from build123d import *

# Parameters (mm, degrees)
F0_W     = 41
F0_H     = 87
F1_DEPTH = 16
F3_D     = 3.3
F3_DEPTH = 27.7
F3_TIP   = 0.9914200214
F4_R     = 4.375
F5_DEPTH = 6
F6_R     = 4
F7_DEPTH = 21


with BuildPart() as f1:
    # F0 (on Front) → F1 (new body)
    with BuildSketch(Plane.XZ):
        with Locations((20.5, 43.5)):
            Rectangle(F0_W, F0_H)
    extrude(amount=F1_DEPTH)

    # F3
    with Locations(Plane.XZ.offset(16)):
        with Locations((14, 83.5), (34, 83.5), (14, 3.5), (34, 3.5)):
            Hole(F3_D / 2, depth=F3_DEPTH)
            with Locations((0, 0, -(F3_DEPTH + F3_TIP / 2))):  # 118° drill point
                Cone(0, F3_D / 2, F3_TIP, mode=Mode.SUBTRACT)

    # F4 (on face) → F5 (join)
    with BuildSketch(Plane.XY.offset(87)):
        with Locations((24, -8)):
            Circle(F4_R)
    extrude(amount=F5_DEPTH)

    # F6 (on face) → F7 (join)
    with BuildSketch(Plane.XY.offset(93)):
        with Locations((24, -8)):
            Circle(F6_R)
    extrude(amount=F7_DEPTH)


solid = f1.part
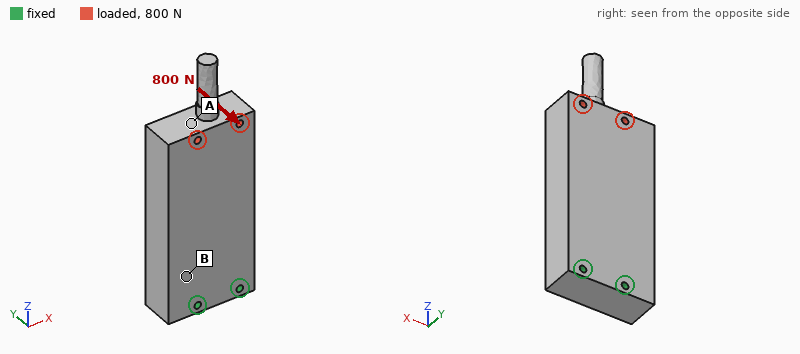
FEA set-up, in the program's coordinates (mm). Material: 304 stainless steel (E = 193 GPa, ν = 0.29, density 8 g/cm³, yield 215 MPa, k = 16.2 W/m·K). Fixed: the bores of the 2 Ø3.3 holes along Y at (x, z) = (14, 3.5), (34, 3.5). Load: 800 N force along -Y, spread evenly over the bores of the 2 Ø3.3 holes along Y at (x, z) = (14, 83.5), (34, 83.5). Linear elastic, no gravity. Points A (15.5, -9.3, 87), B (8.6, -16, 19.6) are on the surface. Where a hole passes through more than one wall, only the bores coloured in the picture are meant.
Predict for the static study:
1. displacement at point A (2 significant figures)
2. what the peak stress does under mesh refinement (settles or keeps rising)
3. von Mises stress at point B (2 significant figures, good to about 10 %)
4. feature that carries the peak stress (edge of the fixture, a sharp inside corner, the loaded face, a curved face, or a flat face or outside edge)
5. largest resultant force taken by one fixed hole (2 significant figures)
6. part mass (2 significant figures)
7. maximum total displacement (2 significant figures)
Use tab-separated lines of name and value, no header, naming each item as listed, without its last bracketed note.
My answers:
displacement at point A	66 µm
what the peak stress does under mesh refinement	keeps rising
von Mises stress at point B	27 MPa
feature that carries the peak stress	edge of the fixture
largest resultant force taken by one fixed hole	410 N
part mass	460 g
maximum total displacement	96 µm
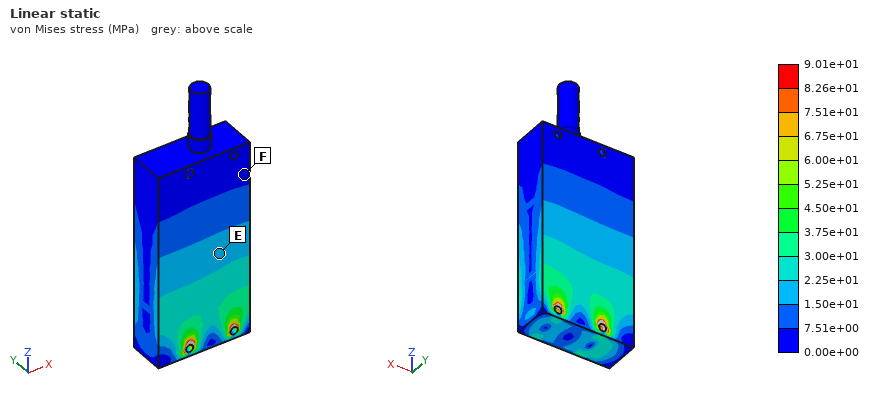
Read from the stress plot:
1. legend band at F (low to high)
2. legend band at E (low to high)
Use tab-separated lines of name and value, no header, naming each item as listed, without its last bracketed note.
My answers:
legend band at F	0.00e+00 to 7.51e+00 MPa
legend band at E	1.50e+01 to 2.25e+01 MPa
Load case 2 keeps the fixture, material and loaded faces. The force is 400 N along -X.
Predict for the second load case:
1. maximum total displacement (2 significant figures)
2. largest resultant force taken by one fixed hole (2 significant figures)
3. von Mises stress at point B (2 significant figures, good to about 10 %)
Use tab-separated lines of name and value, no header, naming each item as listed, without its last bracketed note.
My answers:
maximum total displacement	10 µm
largest resultant force taken by one fixed hole	1.5 kN
von Mises stress at point B	3.9 MPa
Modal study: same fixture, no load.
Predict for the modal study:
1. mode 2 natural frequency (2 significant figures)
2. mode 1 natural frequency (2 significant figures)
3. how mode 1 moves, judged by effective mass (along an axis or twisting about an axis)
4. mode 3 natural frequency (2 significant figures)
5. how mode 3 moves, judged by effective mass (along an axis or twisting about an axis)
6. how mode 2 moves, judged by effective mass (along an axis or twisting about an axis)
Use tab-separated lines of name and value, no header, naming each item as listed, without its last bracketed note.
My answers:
mode 2 natural frequency	3000 Hz
mode 1 natural frequency	1500 Hz
how mode 1 moves, judged by effective mass	along Y
mode 3 natural frequency	5900 Hz
how mode 3 moves, judged by effective mass	twisting about Z
how mode 2 moves, judged by effective mass	along X
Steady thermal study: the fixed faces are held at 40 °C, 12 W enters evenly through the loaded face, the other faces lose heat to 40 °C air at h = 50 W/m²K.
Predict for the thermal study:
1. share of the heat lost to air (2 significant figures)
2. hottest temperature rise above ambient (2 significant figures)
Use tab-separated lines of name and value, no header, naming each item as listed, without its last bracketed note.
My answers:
share of the heat lost to air	78 %
hottest temperature rise above ambient	44 K
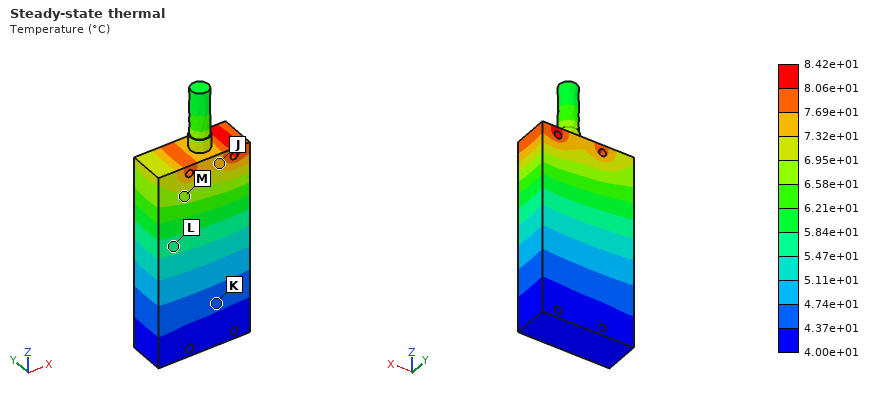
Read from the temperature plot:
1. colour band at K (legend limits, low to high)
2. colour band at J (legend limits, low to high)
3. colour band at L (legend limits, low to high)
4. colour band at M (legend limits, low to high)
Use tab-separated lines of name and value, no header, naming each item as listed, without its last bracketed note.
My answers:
colour band at K	4.37e+01 to 4.74e+01 °C
colour band at J	7.32e+01 to 7.69e+01 °C
colour band at L	5.47e+01 to 5.84e+01 °C
colour band at M	6.58e+01 to 6.95e+01 °C
